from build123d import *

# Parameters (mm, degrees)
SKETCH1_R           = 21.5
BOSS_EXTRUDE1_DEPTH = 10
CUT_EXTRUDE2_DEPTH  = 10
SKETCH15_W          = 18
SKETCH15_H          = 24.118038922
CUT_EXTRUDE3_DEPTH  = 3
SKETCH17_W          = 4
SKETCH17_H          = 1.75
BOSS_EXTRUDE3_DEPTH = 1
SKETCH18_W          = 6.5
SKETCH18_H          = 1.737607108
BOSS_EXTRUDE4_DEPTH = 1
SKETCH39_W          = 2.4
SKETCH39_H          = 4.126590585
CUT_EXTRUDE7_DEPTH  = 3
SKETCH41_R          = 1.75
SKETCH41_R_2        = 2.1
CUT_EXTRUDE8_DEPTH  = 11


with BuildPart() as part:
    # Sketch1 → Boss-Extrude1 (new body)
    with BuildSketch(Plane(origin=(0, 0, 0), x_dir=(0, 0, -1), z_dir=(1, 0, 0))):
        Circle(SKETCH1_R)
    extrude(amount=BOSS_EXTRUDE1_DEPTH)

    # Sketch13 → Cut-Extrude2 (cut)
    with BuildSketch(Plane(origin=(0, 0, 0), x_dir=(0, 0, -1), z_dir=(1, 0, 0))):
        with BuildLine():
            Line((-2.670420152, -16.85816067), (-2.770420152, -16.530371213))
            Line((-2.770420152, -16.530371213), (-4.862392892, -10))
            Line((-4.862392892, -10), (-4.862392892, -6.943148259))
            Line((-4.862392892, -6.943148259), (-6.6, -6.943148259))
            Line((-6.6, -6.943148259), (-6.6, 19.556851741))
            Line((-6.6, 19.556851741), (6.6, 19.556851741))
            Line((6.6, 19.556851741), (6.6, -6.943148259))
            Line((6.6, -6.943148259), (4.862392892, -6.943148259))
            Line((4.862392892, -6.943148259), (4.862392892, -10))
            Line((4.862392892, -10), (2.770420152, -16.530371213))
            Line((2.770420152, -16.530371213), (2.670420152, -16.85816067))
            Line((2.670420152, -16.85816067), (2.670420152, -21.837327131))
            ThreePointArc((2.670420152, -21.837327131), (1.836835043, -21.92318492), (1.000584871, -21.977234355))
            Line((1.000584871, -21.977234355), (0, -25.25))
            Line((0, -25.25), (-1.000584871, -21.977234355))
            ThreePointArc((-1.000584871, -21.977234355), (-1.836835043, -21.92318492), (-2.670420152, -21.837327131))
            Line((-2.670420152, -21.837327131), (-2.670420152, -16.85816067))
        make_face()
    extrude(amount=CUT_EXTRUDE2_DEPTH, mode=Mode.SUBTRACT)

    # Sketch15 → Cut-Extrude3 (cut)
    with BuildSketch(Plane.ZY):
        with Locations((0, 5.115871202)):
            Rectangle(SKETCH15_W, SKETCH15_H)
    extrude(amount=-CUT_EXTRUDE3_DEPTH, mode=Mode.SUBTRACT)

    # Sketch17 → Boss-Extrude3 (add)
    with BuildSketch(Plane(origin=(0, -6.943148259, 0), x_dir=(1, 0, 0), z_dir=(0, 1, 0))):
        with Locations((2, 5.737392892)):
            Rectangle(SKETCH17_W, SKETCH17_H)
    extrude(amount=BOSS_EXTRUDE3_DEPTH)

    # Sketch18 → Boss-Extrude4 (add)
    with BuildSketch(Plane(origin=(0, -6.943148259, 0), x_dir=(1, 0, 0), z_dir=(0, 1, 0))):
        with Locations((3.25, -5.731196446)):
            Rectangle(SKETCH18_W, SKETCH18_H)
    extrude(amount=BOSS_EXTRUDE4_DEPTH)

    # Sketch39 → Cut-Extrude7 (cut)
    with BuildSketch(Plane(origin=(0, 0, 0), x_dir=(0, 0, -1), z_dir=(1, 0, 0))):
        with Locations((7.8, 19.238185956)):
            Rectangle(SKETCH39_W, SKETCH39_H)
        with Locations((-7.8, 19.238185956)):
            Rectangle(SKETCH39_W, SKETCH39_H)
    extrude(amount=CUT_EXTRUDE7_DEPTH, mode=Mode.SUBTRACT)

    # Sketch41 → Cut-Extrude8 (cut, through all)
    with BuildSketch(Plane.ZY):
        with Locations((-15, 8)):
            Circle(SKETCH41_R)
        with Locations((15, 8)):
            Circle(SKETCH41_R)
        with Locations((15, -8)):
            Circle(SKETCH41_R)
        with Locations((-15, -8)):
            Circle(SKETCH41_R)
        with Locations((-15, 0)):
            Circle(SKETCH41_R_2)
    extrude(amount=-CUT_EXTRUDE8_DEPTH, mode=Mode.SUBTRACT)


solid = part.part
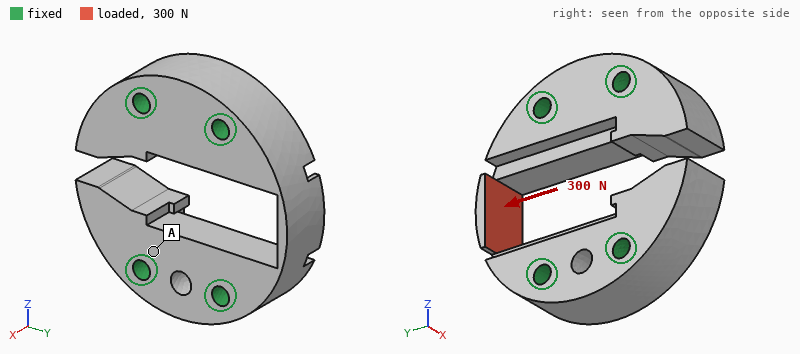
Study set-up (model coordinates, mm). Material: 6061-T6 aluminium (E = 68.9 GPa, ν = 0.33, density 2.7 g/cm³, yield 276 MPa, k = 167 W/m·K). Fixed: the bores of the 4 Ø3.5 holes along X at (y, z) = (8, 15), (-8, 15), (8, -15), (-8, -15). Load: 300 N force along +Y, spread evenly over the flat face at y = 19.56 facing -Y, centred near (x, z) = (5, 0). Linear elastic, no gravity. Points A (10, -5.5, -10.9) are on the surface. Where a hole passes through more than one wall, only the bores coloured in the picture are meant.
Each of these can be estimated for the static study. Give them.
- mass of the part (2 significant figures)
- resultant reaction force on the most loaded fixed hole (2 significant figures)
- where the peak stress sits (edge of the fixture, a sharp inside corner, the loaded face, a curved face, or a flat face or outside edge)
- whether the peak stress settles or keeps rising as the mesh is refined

24 g
210 N
a sharp inside corner
keeps rising
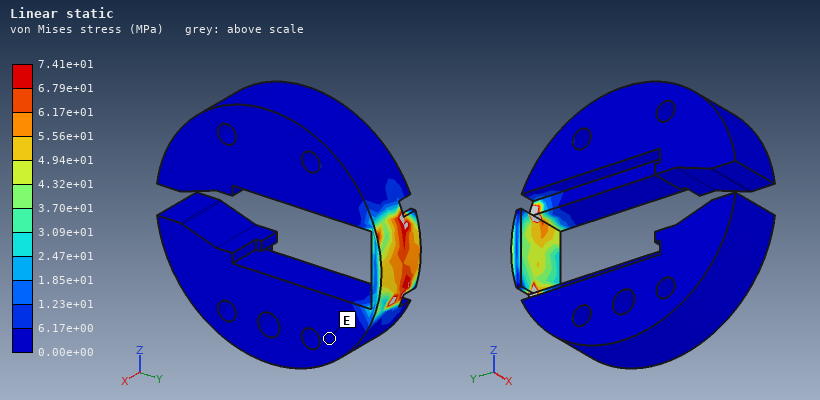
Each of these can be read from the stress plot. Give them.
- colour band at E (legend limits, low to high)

0.00e+00 to 6.17e+00 MPa
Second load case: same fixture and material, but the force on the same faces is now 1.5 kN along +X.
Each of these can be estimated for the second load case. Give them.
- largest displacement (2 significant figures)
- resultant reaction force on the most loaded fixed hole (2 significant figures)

46 µm
840 N
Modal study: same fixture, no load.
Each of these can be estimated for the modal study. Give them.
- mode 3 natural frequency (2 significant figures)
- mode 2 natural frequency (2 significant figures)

30 kHz
29 kHz
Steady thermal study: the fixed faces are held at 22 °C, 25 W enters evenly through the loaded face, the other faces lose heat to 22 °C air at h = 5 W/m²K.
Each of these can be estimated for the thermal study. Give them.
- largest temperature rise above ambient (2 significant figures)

55 K
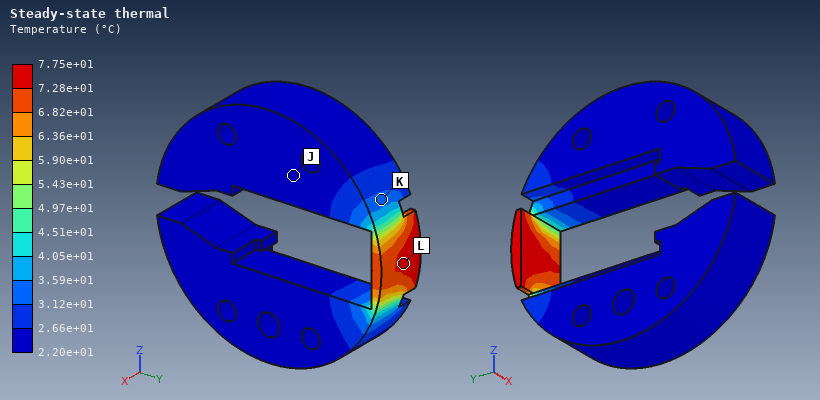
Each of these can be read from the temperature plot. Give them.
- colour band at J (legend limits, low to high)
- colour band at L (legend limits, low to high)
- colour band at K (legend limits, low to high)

2.20e+01 to 2.66e+01 °C
7.28e+01 to 7.75e+01 °C
3.12e+01 to 3.59e+01 °C
